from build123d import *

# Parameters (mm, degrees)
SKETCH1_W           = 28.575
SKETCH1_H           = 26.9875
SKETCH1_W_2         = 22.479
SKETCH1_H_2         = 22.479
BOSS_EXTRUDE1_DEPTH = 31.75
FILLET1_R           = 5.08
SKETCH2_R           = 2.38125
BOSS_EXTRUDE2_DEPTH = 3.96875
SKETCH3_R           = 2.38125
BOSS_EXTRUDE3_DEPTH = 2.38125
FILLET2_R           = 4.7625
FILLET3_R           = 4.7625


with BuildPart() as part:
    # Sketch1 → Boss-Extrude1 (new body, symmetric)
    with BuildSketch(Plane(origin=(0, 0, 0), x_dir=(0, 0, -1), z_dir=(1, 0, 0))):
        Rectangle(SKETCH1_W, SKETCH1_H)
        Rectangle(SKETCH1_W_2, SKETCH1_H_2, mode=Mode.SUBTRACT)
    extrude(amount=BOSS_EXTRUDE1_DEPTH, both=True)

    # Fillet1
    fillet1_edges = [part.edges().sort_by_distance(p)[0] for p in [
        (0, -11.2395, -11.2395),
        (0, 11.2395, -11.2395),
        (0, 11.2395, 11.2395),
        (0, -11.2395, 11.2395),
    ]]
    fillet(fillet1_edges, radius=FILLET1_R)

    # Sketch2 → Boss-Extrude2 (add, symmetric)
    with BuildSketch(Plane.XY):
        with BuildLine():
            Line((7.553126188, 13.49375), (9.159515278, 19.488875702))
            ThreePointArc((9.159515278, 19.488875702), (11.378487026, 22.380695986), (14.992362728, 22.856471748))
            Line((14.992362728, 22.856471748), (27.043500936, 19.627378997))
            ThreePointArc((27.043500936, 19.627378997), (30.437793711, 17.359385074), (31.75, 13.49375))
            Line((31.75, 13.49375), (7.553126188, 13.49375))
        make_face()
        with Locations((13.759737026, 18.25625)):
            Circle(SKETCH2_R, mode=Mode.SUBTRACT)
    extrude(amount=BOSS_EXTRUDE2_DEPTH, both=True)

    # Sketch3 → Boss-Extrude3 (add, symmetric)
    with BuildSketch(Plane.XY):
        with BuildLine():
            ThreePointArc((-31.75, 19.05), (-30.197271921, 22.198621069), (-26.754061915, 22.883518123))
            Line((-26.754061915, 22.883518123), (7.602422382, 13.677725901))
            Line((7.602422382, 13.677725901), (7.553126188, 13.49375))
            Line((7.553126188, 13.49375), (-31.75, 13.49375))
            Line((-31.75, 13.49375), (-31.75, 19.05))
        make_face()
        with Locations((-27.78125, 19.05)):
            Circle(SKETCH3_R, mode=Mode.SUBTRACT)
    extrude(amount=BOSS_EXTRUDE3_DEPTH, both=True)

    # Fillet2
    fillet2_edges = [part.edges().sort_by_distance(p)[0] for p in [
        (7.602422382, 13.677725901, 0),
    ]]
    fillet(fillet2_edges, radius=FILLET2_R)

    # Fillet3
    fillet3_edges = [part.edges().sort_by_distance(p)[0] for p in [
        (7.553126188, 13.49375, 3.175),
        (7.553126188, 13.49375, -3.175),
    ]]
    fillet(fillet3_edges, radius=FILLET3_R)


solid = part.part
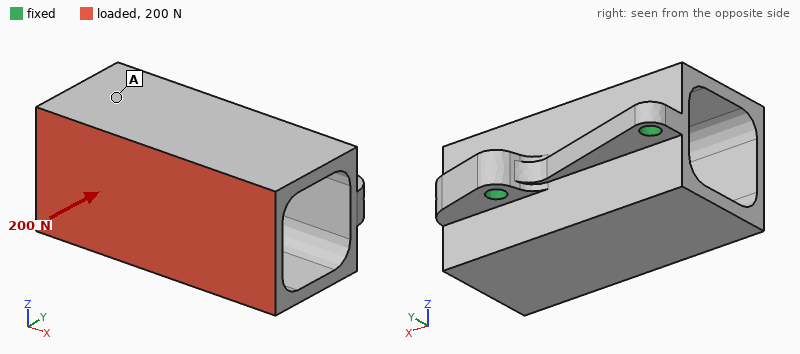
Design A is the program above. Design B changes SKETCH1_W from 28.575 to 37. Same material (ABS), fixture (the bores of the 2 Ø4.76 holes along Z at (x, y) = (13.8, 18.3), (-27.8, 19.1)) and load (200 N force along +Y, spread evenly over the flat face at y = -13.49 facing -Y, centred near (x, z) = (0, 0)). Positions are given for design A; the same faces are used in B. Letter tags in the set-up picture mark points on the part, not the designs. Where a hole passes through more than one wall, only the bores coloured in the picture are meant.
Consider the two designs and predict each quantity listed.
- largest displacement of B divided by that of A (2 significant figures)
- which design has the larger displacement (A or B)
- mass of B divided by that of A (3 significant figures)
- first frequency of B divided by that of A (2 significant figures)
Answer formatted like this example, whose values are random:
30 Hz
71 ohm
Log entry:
0.43
A
1.71
0.75
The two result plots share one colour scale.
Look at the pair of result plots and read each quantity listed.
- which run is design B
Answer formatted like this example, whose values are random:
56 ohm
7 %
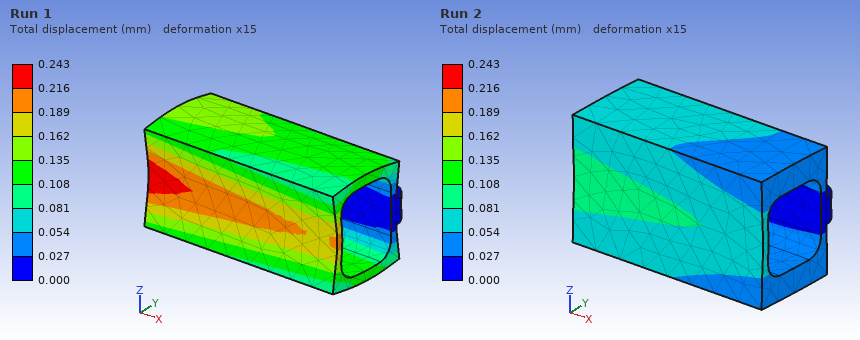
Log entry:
Run 2
